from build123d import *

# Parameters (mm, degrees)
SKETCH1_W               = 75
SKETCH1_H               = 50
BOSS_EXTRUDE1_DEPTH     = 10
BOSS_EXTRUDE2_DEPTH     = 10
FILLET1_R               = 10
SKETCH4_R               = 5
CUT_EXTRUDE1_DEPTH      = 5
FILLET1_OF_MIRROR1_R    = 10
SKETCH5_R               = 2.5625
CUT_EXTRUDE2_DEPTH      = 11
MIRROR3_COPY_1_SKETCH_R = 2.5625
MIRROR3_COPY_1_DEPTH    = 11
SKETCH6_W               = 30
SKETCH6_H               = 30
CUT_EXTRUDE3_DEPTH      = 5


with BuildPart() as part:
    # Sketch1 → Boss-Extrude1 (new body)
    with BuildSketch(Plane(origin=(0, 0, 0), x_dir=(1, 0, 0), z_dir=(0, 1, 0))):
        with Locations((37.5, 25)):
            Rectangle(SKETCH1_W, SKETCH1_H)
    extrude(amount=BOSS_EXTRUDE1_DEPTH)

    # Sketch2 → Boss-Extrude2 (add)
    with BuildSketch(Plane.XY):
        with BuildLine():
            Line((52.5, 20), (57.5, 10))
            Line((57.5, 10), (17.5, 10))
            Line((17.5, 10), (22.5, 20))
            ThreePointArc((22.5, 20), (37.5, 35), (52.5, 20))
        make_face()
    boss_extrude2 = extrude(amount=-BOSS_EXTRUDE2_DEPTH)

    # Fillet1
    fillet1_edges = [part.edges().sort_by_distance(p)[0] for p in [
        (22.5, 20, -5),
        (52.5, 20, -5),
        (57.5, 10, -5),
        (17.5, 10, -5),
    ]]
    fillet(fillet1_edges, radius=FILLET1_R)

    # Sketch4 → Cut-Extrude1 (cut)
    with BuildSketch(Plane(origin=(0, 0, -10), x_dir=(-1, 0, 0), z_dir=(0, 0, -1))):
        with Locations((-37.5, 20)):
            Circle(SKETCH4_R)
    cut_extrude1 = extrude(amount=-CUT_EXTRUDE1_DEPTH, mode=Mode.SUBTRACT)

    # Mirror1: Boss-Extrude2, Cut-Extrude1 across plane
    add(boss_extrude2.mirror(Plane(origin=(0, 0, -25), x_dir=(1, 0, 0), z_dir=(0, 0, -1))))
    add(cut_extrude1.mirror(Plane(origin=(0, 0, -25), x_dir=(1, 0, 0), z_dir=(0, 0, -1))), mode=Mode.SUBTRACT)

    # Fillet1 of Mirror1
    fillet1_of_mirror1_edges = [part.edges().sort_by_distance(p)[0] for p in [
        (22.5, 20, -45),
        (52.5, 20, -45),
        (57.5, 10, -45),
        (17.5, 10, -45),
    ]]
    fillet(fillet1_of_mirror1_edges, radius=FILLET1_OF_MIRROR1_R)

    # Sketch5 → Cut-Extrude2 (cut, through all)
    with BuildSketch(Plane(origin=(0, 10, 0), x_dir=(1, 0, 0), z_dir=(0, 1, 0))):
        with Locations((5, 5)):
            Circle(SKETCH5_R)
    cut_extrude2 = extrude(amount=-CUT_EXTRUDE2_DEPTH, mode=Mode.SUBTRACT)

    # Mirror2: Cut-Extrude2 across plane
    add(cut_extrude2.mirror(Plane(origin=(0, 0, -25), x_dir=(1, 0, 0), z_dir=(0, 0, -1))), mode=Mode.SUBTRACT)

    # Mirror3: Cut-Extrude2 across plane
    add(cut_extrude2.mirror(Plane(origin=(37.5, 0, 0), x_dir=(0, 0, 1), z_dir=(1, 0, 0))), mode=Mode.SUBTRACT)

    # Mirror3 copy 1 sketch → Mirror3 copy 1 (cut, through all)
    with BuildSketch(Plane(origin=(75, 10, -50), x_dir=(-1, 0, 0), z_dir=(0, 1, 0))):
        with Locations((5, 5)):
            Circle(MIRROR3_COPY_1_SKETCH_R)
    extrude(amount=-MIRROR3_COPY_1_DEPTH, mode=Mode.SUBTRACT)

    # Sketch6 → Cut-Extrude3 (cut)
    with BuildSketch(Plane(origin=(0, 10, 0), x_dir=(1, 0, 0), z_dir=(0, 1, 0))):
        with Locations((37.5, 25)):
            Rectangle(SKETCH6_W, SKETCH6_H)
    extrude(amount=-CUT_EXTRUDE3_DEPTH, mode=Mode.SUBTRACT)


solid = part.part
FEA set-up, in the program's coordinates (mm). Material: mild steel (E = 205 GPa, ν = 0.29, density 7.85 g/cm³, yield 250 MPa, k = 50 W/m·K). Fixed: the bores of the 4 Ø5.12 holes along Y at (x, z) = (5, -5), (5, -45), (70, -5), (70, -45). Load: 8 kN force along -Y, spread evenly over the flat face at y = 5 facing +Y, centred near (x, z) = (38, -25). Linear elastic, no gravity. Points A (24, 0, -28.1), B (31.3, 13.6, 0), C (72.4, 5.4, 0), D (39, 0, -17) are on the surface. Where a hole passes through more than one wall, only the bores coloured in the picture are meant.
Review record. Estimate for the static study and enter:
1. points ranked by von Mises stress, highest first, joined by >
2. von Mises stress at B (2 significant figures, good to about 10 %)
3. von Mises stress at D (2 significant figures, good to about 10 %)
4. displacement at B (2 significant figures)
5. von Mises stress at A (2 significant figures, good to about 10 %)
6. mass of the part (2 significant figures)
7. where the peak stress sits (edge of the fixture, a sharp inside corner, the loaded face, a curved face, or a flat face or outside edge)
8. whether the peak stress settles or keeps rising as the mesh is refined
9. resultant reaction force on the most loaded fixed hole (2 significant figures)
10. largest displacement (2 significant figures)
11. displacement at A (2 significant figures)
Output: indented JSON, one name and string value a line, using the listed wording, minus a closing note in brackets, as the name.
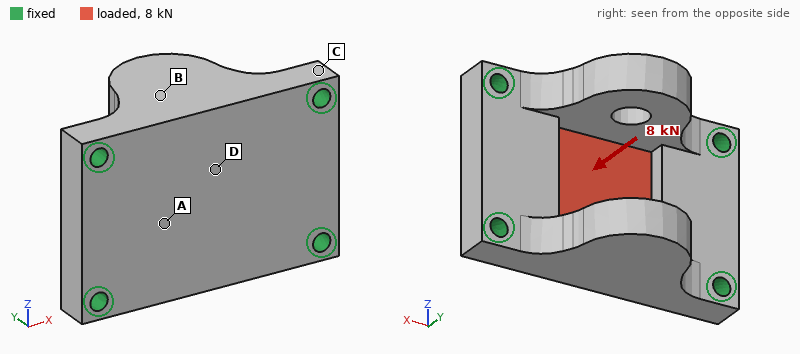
{
  "points ranked by von Mises stress, highest first, joined by >": "D > A > B > C",
  "von Mises stress at B": "23 MPa",
  "von Mises stress at D": "66 MPa",
  "displacement at B": "7.0 µm",
  "von Mises stress at A": "43 MPa",
  "mass of the part": "360 g",
  "where the peak stress sits": "edge of the fixture",
  "whether the peak stress settles or keeps rising as the mesh is refined": "keeps rising",
  "resultant reaction force on the most loaded fixed hole": "2.0 kN",
  "largest displacement": "24 µm",
  "displacement at A": "15 µm"
}
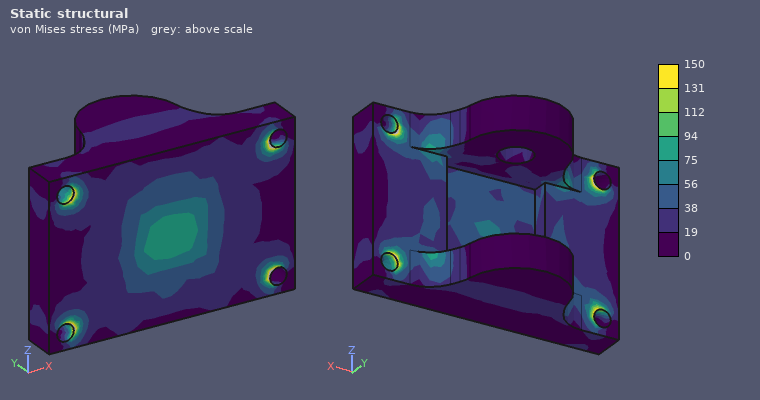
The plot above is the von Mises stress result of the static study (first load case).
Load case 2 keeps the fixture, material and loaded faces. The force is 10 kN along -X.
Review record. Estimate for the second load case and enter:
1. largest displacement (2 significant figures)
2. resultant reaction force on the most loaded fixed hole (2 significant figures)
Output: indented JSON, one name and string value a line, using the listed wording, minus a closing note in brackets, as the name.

{
  "largest displacement": "4.0 µm",
  "resultant reaction force on the most loaded fixed hole": "2.6 kN"
}
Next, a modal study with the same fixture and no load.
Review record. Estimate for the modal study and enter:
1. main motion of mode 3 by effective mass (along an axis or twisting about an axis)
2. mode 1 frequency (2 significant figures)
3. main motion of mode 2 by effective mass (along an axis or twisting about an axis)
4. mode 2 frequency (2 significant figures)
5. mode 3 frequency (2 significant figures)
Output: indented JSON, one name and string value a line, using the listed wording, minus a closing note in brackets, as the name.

{
  "main motion of mode 3 by effective mass": "along Y",
  "mode 1 frequency": "6600 Hz",
  "main motion of mode 2 by effective mass": "along Z",
  "mode 2 frequency": "7000 Hz",
  "mode 3 frequency": "11 kHz"
}
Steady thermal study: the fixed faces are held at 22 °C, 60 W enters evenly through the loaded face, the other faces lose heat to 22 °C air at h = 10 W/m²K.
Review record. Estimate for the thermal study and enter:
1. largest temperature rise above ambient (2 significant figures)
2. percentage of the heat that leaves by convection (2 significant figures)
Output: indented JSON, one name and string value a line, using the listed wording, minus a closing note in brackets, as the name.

{
  "largest temperature rise above ambient": "51 K",
  "percentage of the heat that leaves by convection": "4.3 %"
}
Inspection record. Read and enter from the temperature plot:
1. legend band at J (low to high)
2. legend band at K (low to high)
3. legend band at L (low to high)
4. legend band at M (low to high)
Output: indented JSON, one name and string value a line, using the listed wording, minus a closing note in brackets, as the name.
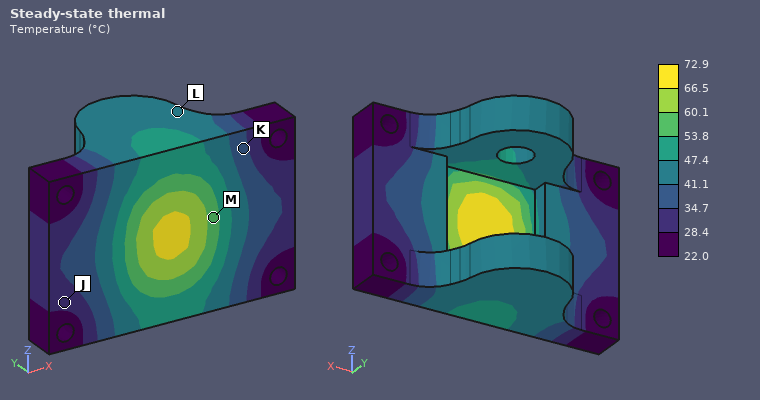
{
  "legend band at J": "28.4 to 34.7 °C",
  "legend band at K": "34.7 to 41.1 °C",
  "legend band at L": "41.1 to 47.4 °C",
  "legend band at M": "53.8 to 60.1 °C"
}
